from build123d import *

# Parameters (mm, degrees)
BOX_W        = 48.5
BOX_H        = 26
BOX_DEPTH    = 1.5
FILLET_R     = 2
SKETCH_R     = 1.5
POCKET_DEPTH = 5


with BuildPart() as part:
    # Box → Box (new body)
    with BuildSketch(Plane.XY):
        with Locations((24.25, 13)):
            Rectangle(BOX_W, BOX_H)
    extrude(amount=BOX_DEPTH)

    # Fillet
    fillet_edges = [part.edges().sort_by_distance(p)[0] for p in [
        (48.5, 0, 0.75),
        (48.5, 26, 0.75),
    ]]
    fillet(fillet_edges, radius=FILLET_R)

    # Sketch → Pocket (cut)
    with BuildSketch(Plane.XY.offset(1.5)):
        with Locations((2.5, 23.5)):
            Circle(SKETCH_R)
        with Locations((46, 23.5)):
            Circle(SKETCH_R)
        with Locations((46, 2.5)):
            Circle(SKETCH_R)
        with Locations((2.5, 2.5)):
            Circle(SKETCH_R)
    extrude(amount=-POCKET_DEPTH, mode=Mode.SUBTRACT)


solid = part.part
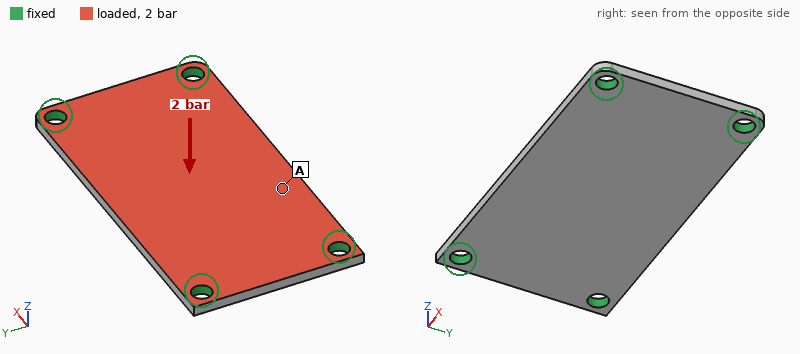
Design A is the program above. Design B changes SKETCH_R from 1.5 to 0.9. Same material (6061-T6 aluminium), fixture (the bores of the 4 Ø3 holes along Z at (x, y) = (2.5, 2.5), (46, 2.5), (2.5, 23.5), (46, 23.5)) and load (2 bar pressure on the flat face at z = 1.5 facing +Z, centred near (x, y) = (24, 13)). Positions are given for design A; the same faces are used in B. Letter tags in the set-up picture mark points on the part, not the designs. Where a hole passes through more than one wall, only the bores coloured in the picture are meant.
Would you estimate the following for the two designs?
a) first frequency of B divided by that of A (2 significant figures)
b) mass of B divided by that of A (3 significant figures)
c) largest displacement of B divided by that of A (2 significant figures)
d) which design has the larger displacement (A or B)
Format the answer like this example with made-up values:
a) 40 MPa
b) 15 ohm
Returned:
a) 0.91
b) 1.01
c) 1.2
d) B
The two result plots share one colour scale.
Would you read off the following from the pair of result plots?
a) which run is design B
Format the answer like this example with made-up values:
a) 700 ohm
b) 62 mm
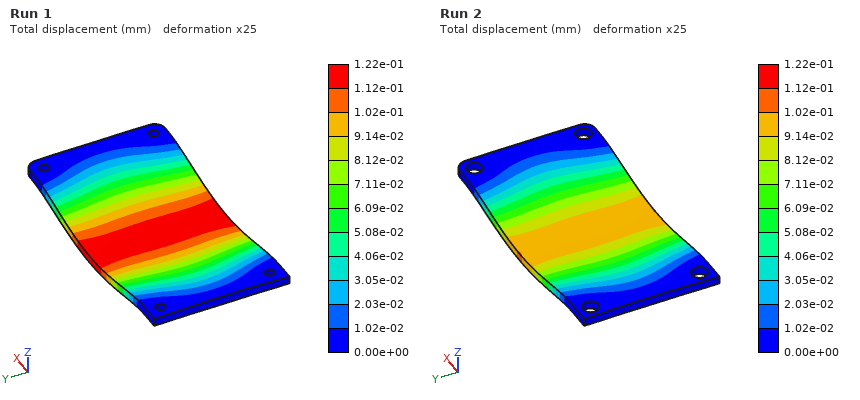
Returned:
a) Run 1
